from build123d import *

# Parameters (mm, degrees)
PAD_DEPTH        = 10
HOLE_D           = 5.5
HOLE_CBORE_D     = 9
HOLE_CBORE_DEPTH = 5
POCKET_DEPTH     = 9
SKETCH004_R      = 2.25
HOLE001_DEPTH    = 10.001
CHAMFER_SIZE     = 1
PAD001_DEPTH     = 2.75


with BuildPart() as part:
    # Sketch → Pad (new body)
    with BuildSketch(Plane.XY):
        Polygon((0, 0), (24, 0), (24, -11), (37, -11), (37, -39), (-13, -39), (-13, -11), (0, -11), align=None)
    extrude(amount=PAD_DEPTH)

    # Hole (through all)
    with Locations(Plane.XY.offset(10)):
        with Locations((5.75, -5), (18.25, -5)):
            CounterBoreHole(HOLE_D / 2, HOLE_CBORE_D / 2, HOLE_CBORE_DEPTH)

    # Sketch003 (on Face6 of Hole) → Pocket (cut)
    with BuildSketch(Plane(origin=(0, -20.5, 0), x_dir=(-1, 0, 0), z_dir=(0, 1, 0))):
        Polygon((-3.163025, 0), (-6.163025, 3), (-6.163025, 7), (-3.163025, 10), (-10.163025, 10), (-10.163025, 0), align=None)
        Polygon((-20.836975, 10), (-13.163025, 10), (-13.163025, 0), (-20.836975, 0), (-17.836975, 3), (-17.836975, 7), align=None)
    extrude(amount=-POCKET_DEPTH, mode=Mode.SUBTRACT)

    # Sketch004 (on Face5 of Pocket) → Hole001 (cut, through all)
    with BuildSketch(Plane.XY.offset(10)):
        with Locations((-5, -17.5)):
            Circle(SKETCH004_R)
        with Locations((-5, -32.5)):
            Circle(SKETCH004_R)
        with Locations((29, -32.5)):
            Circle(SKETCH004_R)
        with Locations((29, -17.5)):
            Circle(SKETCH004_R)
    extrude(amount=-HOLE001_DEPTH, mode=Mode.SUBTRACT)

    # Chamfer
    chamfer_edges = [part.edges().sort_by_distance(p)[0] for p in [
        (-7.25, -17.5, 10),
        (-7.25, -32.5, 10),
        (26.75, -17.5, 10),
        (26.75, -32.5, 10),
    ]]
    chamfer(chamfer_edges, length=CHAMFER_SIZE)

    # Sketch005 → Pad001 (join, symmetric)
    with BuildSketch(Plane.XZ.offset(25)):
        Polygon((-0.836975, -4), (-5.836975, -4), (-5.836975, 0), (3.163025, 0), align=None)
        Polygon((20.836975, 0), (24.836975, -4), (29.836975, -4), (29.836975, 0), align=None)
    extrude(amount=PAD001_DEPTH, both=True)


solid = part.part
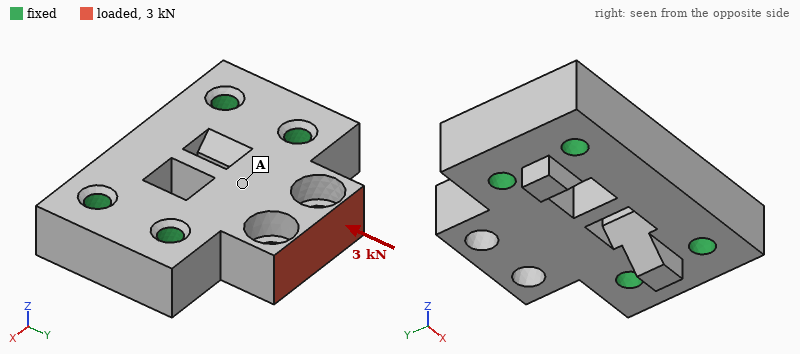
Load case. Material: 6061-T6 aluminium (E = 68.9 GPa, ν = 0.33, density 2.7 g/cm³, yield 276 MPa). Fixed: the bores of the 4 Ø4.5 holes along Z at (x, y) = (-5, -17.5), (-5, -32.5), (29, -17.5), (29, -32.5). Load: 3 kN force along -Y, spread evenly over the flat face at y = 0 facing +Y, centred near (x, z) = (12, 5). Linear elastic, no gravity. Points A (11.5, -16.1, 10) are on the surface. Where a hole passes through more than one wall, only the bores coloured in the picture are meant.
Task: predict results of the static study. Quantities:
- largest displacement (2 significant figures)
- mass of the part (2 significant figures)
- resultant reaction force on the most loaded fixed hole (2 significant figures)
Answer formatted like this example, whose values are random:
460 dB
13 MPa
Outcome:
29 µm
39 g
1.0 kN
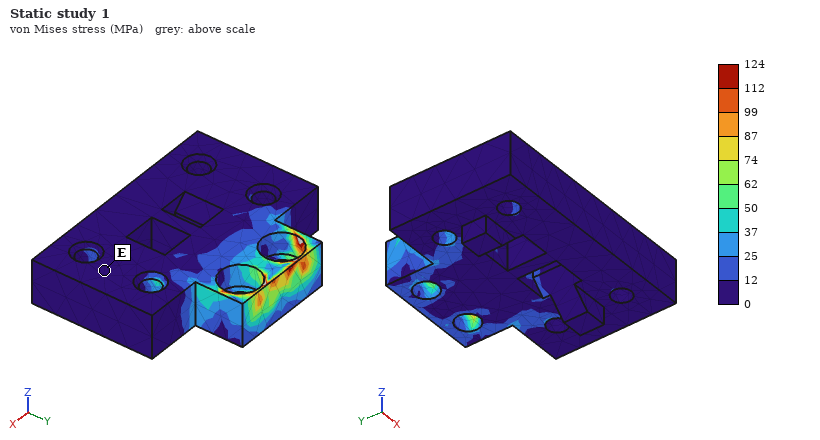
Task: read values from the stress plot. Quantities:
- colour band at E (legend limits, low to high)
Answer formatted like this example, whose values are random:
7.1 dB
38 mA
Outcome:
0 to 12 MPa
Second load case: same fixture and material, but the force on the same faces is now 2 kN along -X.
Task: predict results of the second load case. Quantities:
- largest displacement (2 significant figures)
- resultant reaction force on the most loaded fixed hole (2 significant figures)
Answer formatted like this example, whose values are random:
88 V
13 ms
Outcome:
35 µm
1.3 kN
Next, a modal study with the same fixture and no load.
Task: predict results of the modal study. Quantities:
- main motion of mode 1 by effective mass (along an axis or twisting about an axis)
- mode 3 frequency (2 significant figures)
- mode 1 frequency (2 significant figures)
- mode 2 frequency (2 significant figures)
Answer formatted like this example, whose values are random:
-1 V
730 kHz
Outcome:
along Z
32 kHz
18 kHz
31 kHz
